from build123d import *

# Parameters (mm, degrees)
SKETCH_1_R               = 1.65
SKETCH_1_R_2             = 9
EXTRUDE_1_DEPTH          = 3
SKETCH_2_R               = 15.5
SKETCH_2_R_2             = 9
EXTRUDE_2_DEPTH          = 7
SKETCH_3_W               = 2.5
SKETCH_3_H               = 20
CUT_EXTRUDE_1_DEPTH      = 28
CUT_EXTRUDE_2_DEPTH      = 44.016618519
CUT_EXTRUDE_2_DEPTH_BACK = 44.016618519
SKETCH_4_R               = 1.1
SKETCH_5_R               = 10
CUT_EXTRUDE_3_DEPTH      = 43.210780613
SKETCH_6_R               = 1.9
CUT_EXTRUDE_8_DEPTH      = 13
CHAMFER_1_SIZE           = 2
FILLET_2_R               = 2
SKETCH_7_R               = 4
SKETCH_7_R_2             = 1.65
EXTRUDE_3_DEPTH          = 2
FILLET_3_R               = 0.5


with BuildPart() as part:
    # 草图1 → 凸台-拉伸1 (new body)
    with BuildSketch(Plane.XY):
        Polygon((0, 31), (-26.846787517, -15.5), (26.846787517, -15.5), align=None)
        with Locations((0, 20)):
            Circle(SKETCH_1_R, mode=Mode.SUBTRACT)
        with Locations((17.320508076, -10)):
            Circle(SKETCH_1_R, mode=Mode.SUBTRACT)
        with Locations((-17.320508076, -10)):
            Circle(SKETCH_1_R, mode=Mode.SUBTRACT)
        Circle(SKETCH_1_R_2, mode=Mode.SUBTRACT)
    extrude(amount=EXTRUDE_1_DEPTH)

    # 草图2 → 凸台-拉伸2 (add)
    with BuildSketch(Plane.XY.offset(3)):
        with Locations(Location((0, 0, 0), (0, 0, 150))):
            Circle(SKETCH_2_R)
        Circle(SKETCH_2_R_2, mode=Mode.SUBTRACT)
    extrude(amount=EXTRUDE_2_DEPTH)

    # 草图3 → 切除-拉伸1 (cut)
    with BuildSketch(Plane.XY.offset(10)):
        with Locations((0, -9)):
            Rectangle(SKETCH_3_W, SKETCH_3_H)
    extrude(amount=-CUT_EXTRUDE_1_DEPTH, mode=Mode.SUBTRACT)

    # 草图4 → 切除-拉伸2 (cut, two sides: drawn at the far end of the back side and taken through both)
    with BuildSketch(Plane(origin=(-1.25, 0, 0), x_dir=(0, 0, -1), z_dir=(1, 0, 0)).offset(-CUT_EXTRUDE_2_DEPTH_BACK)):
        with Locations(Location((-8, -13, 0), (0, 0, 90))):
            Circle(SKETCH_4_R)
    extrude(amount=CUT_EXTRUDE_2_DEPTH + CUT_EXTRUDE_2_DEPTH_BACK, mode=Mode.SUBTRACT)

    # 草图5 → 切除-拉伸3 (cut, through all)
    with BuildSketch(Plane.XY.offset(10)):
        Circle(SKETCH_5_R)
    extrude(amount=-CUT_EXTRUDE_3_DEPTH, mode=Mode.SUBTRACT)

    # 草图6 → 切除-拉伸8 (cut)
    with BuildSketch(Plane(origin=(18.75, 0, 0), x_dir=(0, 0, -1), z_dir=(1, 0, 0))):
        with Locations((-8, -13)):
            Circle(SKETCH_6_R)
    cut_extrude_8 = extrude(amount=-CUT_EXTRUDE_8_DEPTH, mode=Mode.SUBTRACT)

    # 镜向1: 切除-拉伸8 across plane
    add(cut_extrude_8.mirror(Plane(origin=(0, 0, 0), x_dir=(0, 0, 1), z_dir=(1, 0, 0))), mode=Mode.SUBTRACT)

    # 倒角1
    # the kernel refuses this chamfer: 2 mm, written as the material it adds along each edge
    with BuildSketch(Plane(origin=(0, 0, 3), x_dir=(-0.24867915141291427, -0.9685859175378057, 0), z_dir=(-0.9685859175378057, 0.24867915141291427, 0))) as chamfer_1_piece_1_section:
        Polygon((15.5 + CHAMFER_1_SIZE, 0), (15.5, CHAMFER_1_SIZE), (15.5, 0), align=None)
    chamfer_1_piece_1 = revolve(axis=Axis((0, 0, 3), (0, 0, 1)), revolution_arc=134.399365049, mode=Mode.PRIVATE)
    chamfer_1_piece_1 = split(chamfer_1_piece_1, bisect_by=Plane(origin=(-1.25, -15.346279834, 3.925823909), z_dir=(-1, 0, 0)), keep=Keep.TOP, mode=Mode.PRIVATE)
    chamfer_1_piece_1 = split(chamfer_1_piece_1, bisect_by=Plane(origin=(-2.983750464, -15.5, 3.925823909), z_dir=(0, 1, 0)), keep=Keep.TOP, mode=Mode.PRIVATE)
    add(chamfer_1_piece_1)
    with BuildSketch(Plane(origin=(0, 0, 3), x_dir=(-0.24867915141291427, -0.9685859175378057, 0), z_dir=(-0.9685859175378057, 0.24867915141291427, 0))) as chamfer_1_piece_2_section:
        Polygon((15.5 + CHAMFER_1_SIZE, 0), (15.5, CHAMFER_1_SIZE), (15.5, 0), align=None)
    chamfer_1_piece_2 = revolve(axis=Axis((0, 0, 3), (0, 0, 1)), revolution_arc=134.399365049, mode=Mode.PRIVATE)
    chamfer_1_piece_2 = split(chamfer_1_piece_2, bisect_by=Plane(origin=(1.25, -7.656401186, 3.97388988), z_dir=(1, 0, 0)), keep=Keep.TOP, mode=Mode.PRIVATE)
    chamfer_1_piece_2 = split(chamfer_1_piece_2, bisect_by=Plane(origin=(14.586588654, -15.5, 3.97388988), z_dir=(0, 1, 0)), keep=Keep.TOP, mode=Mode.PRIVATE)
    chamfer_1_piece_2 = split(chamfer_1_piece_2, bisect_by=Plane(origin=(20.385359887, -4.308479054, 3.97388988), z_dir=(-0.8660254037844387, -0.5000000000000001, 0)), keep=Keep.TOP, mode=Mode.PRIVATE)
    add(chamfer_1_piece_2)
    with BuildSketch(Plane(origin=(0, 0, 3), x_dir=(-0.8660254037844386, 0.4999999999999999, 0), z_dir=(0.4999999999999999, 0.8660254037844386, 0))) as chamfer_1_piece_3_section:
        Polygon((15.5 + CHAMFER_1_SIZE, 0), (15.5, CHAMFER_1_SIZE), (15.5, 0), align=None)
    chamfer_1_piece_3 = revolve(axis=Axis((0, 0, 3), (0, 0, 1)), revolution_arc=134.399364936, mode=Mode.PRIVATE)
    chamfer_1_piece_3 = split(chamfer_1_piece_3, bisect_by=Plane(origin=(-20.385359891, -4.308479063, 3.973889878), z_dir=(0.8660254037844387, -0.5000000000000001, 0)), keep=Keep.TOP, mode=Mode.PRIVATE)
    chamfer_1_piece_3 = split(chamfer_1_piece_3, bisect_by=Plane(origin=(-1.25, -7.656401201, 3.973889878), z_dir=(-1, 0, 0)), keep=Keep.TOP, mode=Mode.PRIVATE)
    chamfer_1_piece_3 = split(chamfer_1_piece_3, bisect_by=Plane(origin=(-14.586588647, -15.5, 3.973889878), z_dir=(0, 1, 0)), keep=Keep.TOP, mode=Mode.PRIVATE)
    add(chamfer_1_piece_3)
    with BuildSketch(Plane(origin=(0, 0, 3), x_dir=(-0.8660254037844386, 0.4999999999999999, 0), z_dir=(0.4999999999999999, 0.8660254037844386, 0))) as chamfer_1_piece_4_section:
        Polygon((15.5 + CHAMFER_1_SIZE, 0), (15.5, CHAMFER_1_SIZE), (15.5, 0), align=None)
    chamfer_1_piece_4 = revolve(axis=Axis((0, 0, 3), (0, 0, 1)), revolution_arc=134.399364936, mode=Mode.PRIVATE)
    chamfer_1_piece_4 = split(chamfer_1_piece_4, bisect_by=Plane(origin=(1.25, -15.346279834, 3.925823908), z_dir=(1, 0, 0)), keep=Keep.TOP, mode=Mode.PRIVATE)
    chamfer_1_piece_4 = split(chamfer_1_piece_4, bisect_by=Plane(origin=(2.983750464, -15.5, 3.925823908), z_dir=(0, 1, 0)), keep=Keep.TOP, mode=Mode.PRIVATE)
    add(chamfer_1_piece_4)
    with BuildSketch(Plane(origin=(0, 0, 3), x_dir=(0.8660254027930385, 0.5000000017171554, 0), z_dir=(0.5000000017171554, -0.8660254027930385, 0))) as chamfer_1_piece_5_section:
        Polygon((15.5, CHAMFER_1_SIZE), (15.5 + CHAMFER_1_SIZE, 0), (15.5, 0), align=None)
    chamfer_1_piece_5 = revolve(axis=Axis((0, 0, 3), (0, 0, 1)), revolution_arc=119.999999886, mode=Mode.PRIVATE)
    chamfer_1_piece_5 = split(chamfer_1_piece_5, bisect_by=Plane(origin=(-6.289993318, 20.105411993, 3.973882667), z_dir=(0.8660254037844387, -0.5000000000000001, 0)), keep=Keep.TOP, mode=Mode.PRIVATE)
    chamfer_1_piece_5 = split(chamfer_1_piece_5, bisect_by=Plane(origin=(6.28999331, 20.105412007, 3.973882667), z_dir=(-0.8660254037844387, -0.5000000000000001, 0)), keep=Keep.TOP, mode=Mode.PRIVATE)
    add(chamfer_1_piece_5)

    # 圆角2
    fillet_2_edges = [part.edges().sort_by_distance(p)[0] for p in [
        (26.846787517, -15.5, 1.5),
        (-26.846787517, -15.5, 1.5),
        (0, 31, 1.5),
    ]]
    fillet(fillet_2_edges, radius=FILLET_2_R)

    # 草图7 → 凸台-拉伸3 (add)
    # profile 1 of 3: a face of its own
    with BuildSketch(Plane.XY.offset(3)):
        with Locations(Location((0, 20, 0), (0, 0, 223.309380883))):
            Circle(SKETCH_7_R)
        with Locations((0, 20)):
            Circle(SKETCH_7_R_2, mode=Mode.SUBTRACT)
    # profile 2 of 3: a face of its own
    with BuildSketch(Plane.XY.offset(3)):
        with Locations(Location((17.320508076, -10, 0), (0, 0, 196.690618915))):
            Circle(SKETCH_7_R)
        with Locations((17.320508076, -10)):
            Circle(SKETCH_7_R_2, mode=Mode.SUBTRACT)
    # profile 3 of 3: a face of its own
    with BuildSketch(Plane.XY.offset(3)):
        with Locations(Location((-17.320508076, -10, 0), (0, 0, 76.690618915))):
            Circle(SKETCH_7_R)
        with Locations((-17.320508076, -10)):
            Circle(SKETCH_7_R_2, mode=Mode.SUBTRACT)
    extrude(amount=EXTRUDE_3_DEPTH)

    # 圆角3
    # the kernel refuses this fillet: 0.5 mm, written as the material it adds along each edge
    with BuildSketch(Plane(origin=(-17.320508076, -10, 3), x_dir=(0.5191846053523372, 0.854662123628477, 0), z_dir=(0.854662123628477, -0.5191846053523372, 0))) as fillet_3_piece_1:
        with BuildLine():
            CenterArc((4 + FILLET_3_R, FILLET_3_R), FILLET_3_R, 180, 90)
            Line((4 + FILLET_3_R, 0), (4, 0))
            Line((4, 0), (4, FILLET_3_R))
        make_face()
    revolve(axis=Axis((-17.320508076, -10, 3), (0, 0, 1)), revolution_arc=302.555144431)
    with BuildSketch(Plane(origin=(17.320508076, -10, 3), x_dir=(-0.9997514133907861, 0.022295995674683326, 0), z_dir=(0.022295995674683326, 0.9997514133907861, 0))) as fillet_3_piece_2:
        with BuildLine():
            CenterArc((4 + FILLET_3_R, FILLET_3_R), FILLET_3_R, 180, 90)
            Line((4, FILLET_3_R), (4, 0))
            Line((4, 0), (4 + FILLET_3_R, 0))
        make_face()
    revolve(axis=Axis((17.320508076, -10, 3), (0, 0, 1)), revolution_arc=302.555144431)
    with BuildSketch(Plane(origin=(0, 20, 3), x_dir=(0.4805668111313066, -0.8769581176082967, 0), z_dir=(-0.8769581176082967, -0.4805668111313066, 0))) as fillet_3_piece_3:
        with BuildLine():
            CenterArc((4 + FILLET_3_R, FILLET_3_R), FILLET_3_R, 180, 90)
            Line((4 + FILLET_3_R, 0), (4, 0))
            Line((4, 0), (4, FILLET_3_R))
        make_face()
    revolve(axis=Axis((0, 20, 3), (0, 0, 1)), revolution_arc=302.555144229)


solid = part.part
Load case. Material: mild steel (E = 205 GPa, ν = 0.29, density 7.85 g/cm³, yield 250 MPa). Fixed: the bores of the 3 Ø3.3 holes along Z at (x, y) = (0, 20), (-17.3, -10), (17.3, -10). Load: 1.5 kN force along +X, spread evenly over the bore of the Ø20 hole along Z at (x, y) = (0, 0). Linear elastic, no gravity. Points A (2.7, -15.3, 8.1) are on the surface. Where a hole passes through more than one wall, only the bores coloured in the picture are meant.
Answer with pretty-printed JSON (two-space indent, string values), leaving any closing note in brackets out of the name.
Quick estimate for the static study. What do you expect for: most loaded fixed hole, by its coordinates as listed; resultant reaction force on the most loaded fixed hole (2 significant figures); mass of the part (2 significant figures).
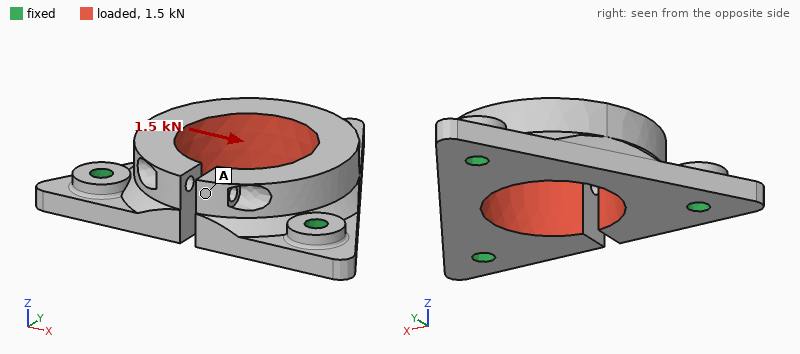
{
  "most loaded fixed hole, by its coordinates as listed": "(0, 20)",
  "resultant reaction force on the most loaded fixed hole": "660 N",
  "mass of the part": "47 g"
}
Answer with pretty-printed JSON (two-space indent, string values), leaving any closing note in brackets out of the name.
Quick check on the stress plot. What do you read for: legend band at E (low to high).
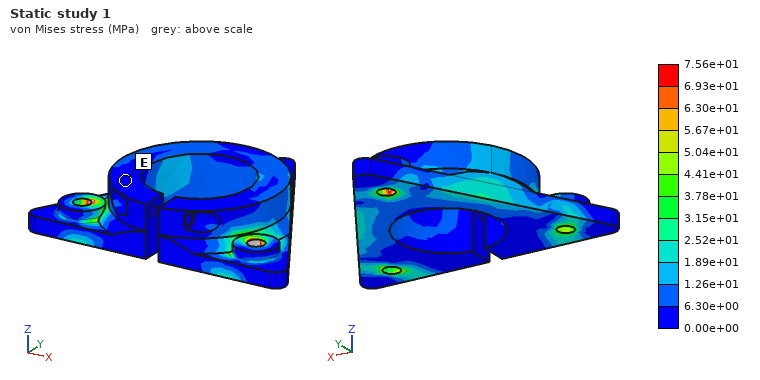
{
  "legend band at E": "0.00e+00 to 6.30e+00 MPa"
}
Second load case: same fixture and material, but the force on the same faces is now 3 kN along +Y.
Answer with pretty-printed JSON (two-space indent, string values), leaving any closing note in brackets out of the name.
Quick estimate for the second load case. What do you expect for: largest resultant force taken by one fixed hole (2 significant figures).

{
  "largest resultant force taken by one fixed hole": "1.1 kN"
}
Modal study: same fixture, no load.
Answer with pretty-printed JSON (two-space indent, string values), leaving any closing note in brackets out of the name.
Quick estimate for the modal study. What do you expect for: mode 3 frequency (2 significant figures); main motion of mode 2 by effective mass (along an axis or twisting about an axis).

{
  "mode 3 frequency": "16 kHz",
  "main motion of mode 2 by effective mass": "along Z"
}
